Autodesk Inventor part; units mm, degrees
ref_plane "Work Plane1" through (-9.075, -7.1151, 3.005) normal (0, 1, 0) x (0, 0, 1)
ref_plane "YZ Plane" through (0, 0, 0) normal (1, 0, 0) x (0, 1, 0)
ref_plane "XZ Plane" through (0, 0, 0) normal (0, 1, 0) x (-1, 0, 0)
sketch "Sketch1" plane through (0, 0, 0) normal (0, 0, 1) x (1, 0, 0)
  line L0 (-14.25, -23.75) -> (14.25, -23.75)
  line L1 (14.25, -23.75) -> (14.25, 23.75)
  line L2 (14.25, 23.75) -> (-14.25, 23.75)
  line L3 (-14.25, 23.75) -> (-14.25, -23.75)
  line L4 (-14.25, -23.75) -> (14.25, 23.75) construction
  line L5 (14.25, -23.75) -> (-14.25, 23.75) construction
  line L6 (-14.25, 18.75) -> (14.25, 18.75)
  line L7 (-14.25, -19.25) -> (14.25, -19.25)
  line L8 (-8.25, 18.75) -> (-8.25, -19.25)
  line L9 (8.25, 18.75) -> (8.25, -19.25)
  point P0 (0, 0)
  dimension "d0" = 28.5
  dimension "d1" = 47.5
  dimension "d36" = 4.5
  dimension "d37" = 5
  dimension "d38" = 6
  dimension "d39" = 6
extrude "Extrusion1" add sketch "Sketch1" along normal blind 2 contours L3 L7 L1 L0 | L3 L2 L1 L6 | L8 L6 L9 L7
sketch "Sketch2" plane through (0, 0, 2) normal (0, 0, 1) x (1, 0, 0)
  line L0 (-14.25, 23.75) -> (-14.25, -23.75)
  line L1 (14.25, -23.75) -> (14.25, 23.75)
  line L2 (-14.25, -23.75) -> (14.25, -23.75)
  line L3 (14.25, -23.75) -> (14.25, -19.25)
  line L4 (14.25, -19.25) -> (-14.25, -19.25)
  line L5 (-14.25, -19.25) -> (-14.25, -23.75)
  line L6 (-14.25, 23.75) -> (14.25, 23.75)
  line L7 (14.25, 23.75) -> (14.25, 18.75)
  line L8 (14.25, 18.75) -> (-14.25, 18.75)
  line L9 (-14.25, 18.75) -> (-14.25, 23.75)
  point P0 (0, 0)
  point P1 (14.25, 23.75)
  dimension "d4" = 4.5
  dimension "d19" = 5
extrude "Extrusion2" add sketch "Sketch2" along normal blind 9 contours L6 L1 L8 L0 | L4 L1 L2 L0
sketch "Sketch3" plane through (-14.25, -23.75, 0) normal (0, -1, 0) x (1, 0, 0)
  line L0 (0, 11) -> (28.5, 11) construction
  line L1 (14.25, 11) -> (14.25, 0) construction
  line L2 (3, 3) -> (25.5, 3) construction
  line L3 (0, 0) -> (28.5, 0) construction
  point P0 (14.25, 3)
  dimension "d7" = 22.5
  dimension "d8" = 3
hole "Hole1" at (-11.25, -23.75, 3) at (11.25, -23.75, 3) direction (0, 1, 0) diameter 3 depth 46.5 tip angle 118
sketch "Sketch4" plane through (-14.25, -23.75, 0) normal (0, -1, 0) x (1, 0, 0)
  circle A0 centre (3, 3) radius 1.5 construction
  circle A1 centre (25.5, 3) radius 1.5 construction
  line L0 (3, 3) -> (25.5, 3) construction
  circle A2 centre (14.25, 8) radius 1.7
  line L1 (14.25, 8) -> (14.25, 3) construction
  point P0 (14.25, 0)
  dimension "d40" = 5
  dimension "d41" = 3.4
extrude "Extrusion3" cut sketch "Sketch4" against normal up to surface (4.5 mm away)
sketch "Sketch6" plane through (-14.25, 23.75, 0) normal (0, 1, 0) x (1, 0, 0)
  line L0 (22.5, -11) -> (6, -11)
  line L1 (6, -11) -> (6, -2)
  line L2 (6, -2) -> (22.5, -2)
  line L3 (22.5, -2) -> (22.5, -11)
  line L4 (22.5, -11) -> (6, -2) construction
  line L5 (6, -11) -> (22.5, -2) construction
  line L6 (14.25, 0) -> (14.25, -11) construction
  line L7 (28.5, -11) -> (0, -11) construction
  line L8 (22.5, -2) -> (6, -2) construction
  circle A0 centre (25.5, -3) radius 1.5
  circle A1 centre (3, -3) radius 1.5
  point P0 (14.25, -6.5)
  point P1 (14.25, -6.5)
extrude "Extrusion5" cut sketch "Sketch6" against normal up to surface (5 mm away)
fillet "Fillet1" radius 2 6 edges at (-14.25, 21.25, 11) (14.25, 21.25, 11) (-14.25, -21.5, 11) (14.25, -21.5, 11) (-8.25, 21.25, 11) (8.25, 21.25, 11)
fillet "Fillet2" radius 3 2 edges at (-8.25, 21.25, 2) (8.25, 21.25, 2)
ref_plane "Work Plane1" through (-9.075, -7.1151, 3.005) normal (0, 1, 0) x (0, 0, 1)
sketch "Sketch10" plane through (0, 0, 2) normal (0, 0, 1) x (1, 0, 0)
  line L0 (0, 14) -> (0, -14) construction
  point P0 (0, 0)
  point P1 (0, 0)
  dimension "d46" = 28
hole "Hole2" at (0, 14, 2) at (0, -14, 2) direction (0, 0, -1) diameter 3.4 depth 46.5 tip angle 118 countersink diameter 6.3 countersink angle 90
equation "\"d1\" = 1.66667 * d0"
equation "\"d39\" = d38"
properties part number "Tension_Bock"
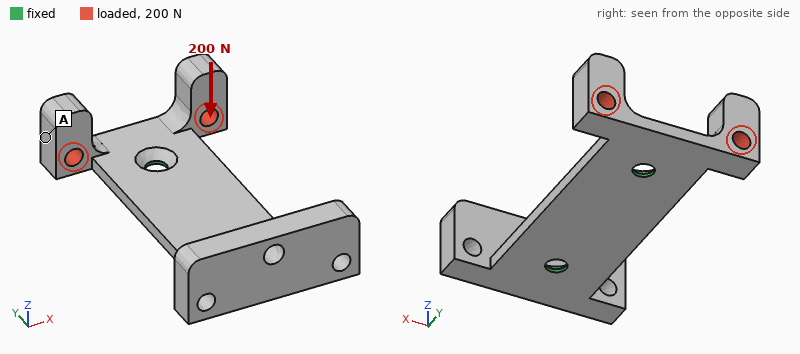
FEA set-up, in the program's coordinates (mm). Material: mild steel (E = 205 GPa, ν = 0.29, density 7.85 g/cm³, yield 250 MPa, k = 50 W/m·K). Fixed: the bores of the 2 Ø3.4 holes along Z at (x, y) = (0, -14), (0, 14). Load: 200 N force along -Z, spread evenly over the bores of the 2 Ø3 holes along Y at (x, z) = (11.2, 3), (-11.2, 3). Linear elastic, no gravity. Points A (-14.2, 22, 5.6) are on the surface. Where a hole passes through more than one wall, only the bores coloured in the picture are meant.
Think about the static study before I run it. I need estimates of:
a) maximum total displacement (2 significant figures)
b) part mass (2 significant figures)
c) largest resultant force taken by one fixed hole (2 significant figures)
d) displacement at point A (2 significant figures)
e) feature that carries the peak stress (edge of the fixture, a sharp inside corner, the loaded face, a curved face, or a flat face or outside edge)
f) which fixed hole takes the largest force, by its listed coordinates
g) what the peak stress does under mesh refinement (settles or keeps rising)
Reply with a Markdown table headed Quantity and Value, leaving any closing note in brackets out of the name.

| Quantity | Value |
|---|---|
| maximum total displacement | 87 µm |
| part mass | 25 g |
| largest resultant force taken by one fixed hole | 300 N |
| displacement at point A | 70 µm |
| feature that carries the peak stress | edge of the fixture |
| which fixed hole takes the largest force, by its listed coordinates | (0, 14) |
| what the peak stress does under mesh refinement | keeps rising |
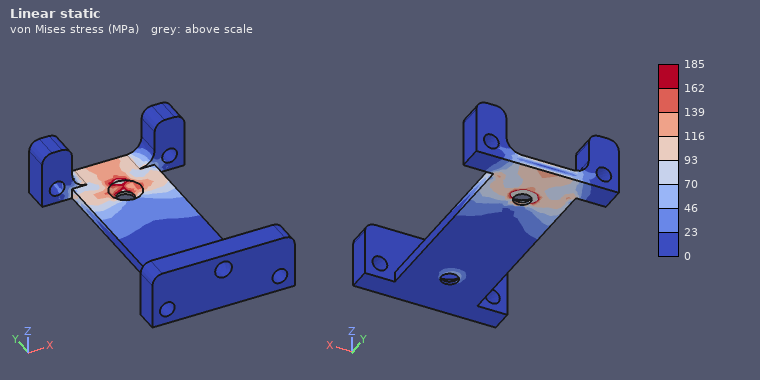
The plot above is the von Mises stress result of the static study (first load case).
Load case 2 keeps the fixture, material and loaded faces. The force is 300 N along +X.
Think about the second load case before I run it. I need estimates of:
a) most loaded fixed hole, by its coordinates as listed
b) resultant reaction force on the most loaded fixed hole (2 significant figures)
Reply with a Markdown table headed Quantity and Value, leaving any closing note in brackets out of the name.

| Quantity | Value |
|---|---|
| most loaded fixed hole, by its coordinates as listed | (0, 14) |
| resultant reaction force on the most loaded fixed hole | 360 N |
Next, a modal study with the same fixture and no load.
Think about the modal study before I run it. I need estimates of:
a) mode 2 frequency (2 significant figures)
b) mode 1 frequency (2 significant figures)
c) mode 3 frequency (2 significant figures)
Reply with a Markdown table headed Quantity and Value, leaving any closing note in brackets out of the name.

| Quantity | Value |
|---|---|
| mode 2 frequency | 3100 Hz |
| mode 1 frequency | 2800 Hz |
| mode 3 frequency | 3200 Hz |
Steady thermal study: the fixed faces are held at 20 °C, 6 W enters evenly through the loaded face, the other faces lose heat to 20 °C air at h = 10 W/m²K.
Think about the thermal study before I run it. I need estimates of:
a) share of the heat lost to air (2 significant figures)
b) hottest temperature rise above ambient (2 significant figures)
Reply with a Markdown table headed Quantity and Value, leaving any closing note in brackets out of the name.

| Quantity | Value |
|---|---|
| share of the heat lost to air | 7.3 % |
| hottest temperature rise above ambient | 54 K |
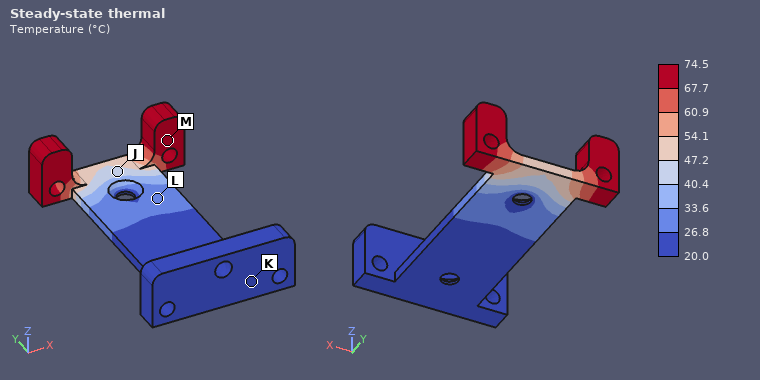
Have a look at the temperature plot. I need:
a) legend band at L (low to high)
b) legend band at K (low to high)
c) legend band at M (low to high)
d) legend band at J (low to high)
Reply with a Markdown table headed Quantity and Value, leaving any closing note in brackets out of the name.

| Quantity | Value |
|---|---|
| legend band at L | 26.8 to 33.6 °C |
| legend band at K | 20.0 to 26.8 °C |
| legend band at M | 67.7 to 74.5 °C |
| legend band at J | 40.4 to 47.2 °C |
